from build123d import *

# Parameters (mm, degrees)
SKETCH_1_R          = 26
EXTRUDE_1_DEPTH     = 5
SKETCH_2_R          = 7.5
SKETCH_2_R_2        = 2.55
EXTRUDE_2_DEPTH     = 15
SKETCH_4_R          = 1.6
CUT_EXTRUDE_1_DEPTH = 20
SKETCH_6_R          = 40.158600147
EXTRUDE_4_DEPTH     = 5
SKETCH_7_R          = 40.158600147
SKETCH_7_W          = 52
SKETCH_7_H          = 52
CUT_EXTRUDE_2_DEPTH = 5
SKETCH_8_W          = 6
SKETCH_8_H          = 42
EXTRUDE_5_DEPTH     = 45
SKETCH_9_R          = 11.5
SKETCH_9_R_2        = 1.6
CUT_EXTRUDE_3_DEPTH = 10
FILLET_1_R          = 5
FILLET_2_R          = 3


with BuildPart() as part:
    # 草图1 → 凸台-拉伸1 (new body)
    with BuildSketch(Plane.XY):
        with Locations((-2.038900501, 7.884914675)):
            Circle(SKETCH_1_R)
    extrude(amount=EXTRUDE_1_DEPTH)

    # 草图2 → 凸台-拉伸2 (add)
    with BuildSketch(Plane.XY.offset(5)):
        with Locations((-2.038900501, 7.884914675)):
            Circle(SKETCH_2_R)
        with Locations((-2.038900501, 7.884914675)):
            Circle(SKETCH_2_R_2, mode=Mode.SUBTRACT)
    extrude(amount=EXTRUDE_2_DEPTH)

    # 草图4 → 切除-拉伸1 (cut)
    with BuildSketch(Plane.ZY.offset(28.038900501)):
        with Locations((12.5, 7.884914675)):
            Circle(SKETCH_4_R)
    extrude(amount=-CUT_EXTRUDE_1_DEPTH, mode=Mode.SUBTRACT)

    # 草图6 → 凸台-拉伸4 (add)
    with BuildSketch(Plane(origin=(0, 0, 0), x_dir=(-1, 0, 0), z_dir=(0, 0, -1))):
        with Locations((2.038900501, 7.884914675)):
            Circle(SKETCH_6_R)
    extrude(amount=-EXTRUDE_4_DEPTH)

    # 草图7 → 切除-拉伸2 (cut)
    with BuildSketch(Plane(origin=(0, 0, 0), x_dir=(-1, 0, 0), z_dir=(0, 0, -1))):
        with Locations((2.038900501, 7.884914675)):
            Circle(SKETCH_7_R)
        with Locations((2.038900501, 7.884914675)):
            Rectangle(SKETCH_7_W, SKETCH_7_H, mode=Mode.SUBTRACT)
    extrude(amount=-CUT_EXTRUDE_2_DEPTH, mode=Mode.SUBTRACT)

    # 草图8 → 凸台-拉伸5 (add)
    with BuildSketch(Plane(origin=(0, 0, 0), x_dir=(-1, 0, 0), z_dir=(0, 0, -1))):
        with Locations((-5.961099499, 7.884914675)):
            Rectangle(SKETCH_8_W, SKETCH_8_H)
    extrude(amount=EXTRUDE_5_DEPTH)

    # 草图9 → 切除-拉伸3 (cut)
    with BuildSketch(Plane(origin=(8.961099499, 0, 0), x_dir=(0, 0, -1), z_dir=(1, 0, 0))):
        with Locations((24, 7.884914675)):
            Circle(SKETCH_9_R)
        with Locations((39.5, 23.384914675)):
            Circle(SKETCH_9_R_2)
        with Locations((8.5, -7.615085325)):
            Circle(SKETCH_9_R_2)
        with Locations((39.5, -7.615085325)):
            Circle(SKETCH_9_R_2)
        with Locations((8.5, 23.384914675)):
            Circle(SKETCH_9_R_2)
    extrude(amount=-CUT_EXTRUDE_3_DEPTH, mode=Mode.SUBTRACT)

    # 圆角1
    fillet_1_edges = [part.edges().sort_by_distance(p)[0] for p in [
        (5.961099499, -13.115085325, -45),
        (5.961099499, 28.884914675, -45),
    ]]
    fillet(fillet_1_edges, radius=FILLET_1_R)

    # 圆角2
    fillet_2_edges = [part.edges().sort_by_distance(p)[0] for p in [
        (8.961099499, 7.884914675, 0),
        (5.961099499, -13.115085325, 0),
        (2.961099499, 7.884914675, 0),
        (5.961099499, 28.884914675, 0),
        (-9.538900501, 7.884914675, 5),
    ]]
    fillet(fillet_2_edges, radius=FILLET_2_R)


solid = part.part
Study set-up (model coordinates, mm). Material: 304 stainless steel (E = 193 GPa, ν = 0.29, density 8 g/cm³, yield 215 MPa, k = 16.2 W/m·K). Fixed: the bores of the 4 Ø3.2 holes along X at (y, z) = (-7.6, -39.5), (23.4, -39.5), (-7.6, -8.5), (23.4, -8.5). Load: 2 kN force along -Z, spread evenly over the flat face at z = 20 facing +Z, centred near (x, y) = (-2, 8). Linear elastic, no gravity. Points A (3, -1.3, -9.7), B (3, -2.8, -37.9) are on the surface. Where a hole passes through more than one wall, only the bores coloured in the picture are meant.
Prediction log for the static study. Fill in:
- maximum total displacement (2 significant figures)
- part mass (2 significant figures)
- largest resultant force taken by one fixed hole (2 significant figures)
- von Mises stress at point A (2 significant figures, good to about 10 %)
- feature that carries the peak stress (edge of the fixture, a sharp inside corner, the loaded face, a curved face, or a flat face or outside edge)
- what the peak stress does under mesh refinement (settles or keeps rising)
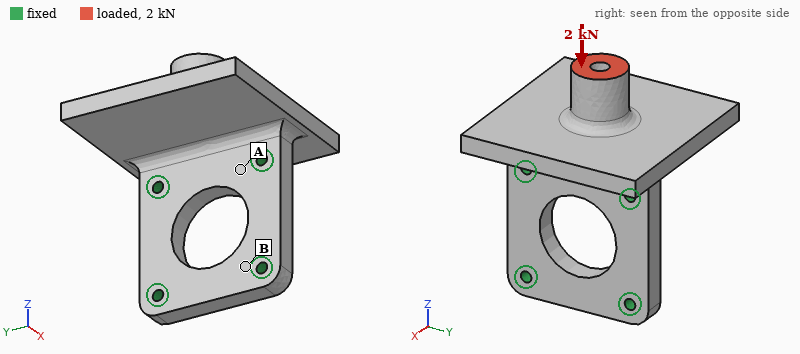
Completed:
52 µm
200 g
1.0 kN
43 MPa
edge of the fixture
keeps rising
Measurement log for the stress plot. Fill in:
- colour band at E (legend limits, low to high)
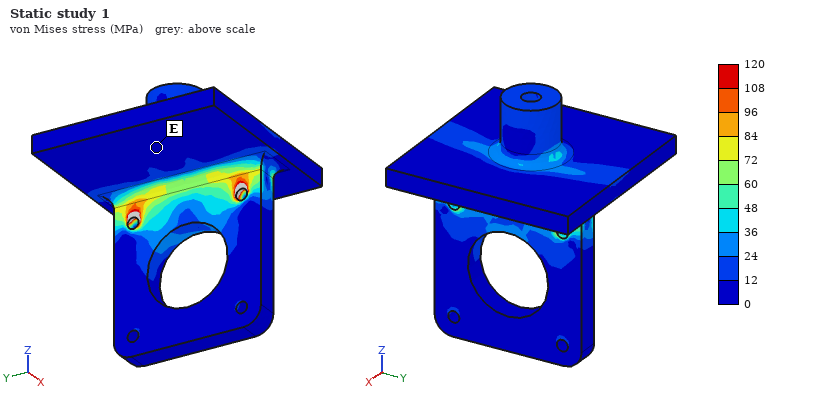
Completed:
0 to 12 MPa
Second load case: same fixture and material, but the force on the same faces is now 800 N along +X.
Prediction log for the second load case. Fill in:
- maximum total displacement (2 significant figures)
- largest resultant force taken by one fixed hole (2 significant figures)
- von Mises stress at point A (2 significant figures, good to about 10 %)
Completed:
65 µm
480 N
45 MPa
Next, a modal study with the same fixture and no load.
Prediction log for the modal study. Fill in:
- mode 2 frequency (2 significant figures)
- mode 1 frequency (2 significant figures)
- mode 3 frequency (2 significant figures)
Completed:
5500 Hz
2500 Hz
7400 Hz
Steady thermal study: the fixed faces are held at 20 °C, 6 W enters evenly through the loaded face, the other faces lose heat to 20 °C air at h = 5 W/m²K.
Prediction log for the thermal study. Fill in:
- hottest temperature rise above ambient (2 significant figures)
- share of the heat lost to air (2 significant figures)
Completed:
62 K
14 %
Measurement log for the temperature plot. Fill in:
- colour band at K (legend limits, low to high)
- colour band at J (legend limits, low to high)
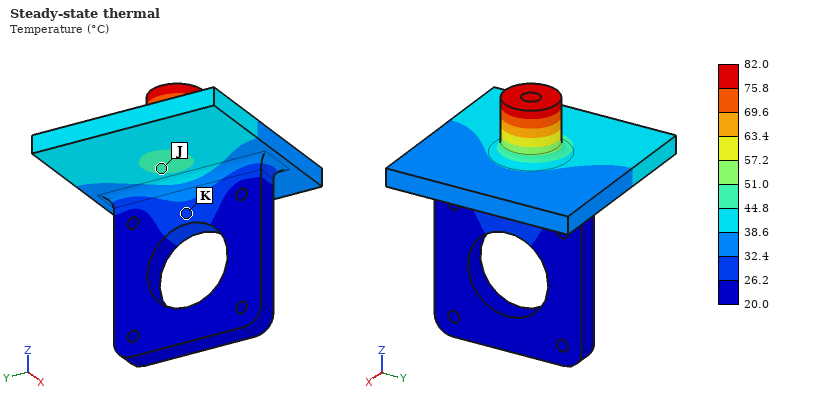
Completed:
26.2 to 32.4 °C
44.8 to 51.0 °C
